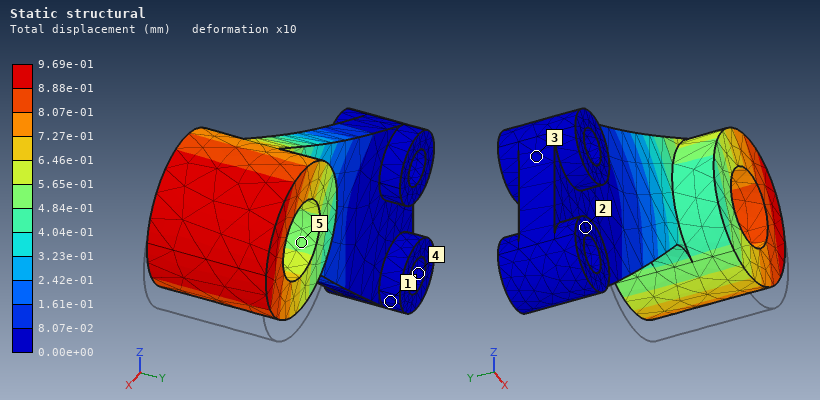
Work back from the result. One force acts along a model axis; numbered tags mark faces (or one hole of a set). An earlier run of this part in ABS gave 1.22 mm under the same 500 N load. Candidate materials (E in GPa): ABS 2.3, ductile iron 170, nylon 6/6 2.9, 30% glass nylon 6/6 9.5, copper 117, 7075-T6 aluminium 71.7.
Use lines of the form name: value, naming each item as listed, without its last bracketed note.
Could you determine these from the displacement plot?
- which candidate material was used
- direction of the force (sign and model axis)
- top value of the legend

which candidate material was used: nylon 6/6
direction of the force: +Z
top value of the legend: 9.69e-01 mm
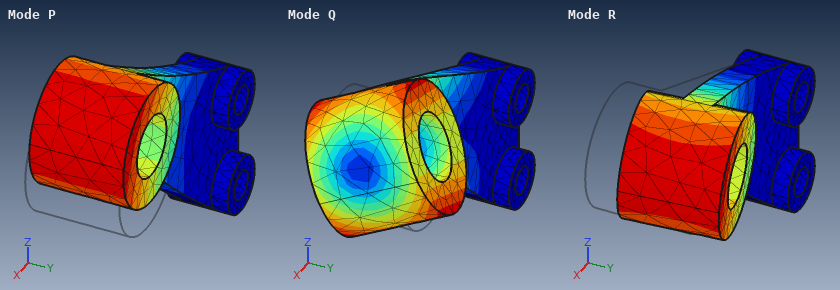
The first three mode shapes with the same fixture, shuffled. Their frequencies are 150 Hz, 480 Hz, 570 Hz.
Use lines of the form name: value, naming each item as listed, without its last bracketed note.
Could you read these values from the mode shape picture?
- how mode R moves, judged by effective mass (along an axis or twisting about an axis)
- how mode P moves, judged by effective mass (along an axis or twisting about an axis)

how mode R moves, judged by effective mass: along Y
how mode P moves, judged by effective mass: along Z
